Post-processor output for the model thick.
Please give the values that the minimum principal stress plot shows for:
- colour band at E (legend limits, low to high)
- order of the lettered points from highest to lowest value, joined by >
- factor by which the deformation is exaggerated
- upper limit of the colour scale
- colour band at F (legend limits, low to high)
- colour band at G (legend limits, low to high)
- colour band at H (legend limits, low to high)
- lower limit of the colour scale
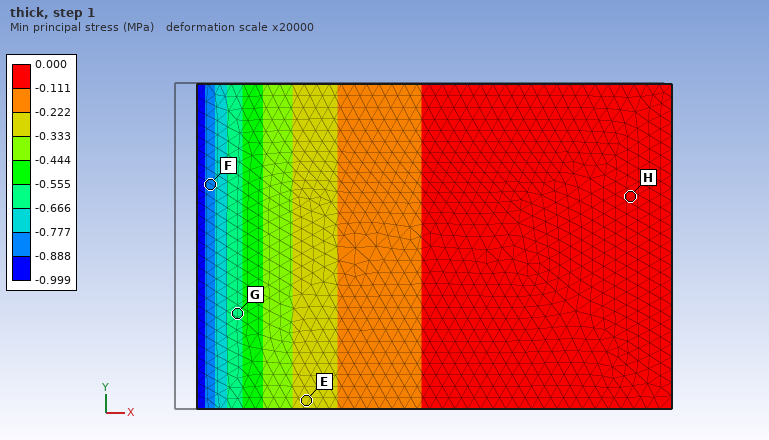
-0.333 to -0.222 MPa
H > E > G > F
20000
0.000 MPa
-0.888 to -0.777 MPa
-0.666 to -0.555 MPa
-0.111 to 0.000 MPa
-0.999 MPa
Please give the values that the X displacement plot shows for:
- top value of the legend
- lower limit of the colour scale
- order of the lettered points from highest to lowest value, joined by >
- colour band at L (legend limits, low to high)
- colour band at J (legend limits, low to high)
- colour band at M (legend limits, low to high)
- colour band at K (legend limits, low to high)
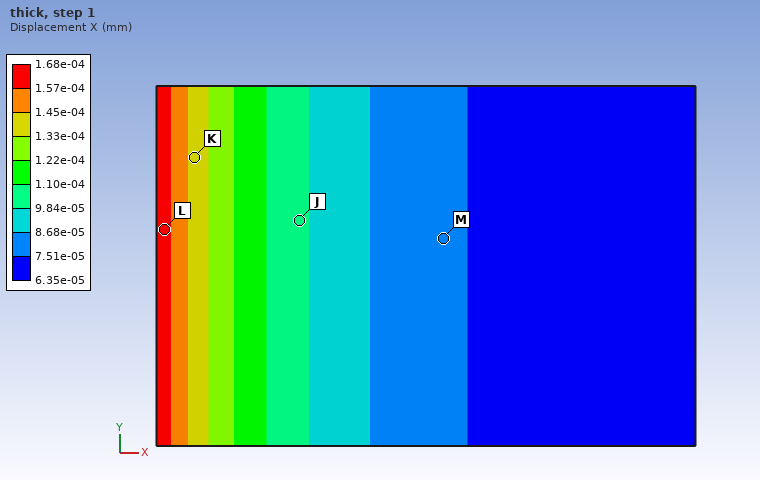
1.68e-04 mm
6.35e-05 mm
L > K > J > M
1.57e-04 to 1.68e-04 mm
9.84e-05 to 1.10e-04 mm
7.51e-05 to 8.68e-05 mm
1.33e-04 to 1.45e-04 mm
